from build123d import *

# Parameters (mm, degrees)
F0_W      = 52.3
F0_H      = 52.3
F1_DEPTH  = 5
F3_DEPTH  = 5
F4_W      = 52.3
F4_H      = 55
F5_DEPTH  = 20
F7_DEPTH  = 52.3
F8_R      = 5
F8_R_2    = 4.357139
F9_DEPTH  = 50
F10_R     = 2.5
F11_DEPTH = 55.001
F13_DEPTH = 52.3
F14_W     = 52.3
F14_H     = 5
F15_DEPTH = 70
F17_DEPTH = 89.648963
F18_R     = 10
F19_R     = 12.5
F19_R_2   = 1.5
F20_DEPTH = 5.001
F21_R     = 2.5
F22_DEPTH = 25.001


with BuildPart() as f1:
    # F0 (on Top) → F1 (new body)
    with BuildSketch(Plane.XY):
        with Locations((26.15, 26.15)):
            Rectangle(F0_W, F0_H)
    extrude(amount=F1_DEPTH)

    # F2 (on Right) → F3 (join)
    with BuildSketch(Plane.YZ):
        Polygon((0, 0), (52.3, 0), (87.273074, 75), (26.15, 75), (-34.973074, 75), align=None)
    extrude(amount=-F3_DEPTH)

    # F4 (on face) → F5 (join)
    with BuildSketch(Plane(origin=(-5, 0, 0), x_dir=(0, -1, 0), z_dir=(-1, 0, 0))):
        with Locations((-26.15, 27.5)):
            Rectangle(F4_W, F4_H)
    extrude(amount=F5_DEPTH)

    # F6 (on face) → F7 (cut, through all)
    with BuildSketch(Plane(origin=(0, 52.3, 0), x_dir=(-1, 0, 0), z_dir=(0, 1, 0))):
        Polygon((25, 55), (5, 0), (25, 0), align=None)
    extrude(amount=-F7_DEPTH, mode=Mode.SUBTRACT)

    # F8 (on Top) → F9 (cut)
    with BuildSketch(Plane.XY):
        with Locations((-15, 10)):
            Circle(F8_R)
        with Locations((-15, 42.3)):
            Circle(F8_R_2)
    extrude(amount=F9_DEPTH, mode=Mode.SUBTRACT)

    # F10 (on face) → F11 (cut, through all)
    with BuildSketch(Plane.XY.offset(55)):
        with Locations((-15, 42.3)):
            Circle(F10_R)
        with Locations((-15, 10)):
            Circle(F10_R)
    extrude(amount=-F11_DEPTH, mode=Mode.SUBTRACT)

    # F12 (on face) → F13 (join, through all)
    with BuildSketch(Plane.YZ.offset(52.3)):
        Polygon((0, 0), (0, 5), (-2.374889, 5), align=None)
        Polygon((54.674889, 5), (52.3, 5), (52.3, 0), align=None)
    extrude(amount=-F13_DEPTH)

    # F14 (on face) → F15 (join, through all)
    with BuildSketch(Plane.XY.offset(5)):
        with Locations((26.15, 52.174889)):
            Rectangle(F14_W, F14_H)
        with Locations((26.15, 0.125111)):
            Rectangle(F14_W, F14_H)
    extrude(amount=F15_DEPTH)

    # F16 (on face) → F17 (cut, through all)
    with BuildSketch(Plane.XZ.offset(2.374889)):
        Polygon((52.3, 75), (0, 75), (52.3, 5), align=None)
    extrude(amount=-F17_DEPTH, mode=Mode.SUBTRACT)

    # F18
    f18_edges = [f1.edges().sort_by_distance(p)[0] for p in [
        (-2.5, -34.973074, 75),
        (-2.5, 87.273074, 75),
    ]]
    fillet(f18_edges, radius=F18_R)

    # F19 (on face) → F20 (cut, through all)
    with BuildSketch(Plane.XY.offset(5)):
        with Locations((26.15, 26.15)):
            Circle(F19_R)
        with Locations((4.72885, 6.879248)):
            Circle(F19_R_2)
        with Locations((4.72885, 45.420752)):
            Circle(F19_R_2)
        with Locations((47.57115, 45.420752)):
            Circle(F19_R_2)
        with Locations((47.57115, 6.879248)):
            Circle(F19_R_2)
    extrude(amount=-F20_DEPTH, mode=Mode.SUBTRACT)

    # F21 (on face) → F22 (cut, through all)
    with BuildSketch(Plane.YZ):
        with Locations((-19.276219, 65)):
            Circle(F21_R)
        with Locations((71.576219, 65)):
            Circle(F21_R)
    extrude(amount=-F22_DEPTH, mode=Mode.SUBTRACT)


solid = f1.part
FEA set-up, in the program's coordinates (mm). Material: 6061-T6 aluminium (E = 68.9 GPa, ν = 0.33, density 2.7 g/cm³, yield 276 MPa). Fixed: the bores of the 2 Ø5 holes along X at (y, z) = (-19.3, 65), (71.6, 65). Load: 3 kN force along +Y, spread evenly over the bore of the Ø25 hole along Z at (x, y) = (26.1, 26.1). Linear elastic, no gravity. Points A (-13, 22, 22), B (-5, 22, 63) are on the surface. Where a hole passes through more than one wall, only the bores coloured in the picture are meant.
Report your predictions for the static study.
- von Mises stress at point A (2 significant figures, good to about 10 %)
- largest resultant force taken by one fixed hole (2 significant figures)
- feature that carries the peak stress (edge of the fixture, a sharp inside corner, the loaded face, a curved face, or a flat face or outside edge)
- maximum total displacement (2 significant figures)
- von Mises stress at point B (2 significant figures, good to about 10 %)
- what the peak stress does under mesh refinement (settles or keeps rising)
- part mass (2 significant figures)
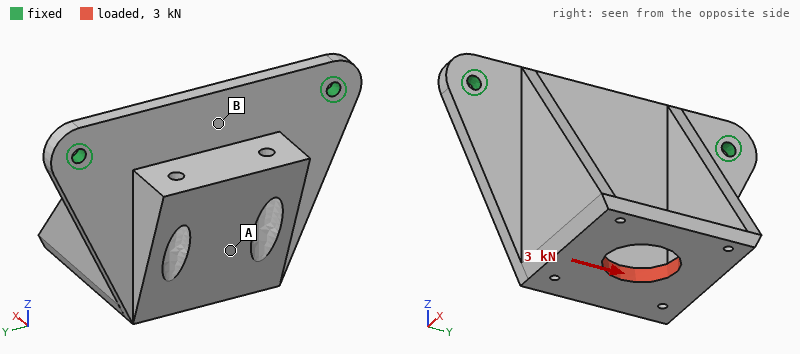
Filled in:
35 MPa
2.8 kN
edge of the fixture
0.45 mm
13 MPa
keeps rising
240 g
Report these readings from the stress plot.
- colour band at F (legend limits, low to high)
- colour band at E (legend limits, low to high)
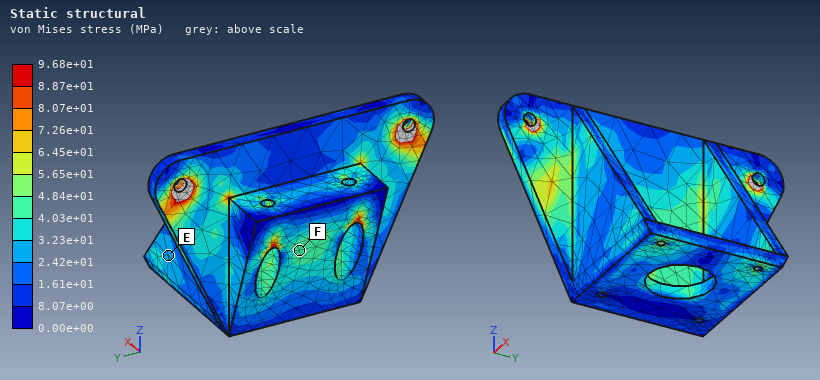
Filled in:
4.03e+01 to 4.84e+01 MPa
2.42e+01 to 3.23e+01 MPa
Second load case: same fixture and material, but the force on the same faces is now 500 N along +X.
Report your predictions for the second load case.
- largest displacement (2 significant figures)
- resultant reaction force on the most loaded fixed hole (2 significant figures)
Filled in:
0.69 mm
250 N
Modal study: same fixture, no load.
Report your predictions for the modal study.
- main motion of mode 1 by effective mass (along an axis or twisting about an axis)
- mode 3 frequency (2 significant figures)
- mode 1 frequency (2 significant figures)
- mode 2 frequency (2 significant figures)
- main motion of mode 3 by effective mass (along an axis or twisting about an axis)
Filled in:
along X
2900 Hz
490 Hz
1800 Hz
along X
